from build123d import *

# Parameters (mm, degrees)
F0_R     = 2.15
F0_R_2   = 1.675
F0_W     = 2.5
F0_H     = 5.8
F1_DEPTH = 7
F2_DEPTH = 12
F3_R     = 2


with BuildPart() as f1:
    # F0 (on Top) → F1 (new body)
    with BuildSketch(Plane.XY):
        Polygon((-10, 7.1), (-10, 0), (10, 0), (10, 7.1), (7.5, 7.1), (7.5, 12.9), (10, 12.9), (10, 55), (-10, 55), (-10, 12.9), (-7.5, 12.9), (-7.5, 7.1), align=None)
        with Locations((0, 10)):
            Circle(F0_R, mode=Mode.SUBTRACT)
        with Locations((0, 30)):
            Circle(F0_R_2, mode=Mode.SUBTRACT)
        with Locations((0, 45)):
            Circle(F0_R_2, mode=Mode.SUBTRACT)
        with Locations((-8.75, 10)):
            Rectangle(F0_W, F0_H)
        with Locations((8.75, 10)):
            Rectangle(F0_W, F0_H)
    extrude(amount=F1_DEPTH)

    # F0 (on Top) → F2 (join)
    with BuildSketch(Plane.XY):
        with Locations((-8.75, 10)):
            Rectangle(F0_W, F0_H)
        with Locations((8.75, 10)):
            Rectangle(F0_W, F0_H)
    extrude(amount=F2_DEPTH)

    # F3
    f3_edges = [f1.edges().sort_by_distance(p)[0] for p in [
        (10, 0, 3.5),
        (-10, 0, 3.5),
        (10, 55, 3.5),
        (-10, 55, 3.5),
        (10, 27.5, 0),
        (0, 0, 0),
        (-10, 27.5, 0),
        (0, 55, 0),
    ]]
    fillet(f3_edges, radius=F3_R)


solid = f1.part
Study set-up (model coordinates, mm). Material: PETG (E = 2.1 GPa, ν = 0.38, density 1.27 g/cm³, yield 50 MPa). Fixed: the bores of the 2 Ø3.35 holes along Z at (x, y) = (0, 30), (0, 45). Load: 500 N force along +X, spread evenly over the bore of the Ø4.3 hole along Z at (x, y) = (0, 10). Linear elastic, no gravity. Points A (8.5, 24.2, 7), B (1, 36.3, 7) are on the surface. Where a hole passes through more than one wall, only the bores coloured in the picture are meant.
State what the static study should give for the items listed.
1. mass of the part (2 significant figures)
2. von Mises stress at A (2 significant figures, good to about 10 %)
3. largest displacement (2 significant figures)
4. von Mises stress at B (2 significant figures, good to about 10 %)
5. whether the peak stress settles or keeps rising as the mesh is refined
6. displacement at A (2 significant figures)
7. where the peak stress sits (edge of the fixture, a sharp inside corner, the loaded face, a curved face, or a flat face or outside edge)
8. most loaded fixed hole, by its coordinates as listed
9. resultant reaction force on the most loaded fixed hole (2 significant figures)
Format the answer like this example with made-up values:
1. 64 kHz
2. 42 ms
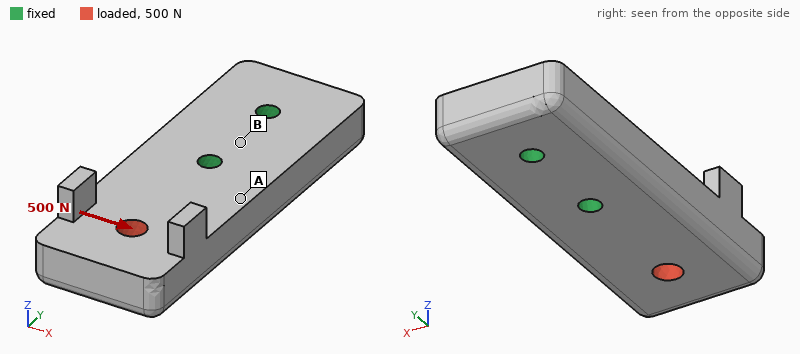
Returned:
1. 9.5 g
2. 14 MPa
3. 0.71 mm
4. 6.1 MPa
5. keeps rising
6. 0.18 mm
7. edge of the fixture
8. (0, 30)
9. 990 N
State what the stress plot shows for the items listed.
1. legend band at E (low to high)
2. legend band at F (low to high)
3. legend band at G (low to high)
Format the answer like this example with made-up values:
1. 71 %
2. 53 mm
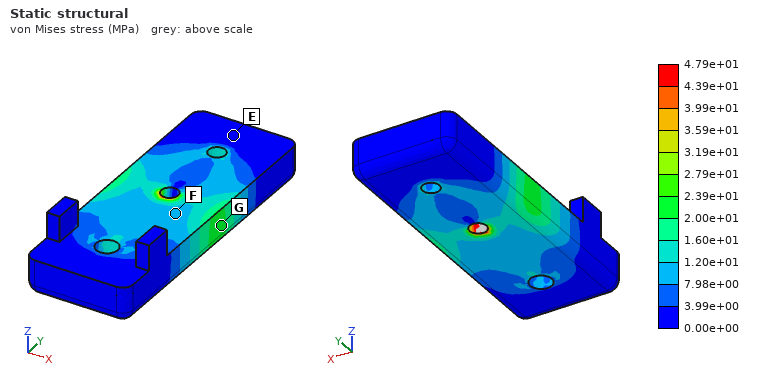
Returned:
1. 0.00e+00 to 3.99e+00 MPa
2. 7.98e+00 to 1.20e+01 MPa
3. 2.00e+01 to 2.39e+01 MPa
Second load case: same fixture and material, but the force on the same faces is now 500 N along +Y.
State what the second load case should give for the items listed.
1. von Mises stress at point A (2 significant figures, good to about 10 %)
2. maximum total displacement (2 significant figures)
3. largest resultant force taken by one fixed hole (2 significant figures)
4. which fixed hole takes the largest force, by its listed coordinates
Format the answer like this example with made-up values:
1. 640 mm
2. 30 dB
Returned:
1. 2.4 MPa
2. 60 µm
3. 390 N
4. (0, 30)
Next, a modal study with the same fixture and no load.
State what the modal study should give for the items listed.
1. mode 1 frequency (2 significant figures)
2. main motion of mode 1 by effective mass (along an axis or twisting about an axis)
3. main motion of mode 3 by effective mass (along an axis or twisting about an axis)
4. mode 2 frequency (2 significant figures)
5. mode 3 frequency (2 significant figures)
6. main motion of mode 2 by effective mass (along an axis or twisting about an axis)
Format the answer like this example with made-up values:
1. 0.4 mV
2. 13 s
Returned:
1. 1500 Hz
2. along Z
3. twisting about Y
4. 2500 Hz
5. 3400 Hz
6. along X
